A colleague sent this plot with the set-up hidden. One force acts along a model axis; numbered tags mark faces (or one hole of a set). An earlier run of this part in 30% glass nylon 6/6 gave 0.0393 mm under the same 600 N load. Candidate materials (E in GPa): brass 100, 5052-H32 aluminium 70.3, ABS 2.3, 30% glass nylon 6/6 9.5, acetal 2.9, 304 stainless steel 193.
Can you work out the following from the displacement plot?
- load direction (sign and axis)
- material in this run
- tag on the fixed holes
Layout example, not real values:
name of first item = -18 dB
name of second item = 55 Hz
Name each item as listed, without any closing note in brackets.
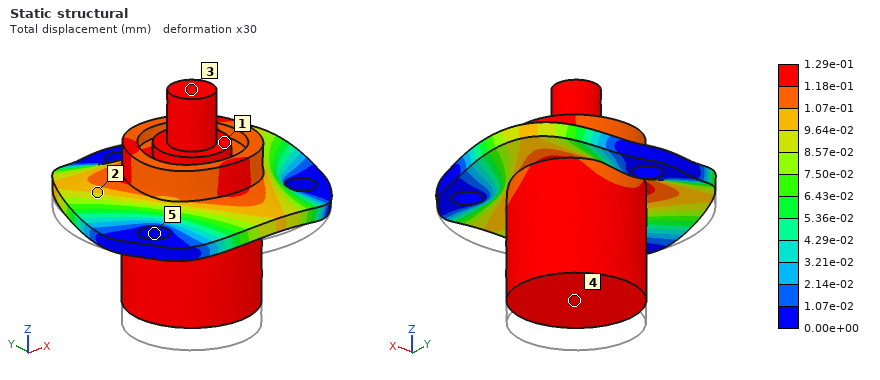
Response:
load direction = +Z
material in this run = acetal
tag on the fixed holes = 5
